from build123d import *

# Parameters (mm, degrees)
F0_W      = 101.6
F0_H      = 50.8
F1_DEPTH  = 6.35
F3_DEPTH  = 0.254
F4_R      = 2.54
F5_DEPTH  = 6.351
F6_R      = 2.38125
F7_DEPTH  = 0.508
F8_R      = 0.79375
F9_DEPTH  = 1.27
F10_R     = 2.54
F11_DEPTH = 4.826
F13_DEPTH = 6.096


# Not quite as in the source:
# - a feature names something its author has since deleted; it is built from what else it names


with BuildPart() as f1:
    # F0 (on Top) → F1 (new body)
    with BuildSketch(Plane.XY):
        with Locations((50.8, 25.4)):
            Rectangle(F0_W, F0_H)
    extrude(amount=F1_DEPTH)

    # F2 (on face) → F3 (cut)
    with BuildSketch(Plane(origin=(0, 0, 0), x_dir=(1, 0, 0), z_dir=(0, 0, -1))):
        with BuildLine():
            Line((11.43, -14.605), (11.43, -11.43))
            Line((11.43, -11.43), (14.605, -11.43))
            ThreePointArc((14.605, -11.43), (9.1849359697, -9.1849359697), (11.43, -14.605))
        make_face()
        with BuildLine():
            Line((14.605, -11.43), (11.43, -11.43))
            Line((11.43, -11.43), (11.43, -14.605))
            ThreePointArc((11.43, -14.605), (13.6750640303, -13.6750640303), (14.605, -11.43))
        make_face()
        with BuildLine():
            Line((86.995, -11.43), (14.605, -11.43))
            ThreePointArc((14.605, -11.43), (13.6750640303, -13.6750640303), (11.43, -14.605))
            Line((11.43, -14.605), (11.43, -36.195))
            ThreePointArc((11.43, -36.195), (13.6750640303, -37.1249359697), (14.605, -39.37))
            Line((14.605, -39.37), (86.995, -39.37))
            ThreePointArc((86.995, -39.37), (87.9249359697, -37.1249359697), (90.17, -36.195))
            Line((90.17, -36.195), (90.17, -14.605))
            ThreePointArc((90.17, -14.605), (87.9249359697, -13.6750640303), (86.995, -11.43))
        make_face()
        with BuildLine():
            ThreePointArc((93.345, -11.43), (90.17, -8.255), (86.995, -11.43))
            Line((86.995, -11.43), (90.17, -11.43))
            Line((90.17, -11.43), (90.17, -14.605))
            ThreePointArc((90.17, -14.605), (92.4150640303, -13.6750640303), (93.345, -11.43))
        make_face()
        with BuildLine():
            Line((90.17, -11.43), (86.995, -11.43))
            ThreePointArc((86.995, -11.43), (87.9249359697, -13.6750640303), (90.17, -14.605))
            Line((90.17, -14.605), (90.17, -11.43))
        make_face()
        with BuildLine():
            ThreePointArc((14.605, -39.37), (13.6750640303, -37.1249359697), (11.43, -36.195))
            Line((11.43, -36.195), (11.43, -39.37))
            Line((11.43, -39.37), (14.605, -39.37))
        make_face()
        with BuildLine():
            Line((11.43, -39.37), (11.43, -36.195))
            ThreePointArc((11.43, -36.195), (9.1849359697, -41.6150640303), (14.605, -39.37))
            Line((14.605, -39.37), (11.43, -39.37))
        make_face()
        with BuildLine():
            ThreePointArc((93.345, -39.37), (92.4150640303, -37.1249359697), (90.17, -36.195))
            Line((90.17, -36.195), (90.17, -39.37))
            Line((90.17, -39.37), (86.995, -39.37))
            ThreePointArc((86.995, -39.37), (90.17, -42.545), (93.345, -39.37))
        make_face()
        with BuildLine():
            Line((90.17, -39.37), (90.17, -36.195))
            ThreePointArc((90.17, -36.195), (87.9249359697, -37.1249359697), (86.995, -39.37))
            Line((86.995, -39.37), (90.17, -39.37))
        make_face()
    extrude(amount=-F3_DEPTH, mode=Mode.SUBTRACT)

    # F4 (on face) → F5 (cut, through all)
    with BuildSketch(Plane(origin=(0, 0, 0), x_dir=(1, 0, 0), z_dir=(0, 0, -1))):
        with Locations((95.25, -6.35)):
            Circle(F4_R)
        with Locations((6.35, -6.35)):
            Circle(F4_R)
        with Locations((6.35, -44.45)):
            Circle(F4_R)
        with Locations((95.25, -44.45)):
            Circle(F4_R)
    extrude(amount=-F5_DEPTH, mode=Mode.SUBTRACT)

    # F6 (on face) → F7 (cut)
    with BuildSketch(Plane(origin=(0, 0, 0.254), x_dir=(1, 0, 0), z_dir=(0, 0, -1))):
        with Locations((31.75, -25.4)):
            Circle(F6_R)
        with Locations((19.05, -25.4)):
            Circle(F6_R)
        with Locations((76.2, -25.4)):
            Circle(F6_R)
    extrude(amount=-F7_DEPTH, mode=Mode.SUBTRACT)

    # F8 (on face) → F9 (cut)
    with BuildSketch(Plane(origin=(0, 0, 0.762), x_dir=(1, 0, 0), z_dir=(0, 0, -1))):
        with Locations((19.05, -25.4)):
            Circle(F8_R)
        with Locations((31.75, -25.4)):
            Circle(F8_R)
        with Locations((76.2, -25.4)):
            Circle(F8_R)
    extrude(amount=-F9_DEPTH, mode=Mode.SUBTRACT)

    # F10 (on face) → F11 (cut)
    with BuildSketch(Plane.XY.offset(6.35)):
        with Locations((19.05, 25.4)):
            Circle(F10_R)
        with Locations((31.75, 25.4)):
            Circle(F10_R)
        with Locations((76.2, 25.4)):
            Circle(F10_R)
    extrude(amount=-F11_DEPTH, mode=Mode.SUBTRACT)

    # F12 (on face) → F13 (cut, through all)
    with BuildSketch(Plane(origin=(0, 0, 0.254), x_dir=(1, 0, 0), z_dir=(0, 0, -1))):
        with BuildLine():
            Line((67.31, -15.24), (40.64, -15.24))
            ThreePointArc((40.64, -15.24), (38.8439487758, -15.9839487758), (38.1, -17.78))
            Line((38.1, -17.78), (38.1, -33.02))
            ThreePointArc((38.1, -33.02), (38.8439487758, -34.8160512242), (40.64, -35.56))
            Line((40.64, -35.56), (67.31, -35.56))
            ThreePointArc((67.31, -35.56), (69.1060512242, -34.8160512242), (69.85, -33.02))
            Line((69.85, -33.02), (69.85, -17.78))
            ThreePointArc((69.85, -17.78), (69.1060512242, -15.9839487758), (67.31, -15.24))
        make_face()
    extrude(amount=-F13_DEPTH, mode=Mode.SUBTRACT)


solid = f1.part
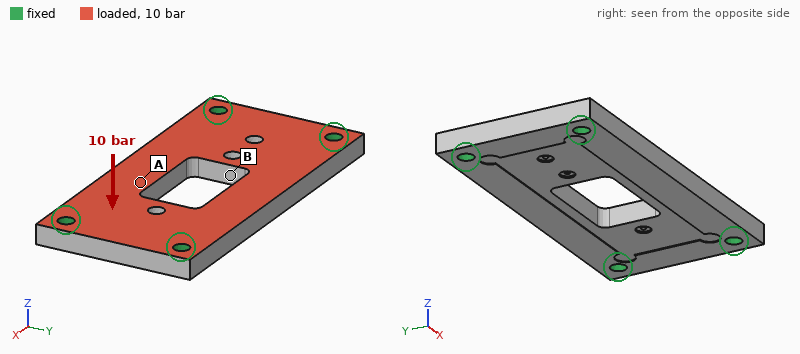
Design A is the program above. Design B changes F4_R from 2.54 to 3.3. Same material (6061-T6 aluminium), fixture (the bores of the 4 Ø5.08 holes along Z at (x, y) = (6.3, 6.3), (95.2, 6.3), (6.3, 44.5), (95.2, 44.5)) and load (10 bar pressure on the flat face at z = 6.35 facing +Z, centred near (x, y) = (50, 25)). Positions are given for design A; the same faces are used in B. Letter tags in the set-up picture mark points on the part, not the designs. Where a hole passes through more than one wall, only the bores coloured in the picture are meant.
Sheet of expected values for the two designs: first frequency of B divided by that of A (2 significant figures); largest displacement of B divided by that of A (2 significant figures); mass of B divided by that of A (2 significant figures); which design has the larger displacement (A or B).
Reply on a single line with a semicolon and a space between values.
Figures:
1.1; 0.89; 0.99; A
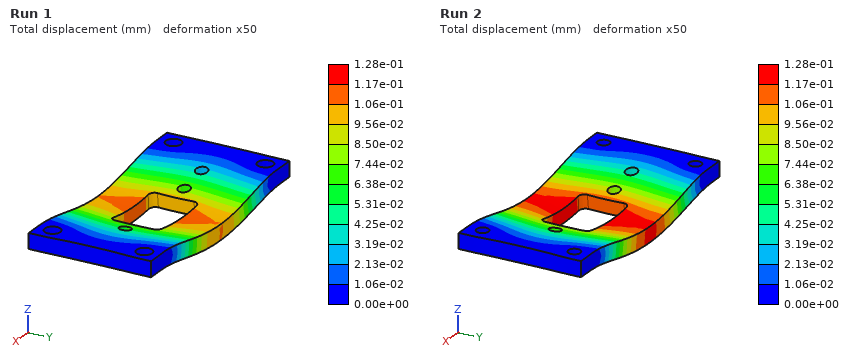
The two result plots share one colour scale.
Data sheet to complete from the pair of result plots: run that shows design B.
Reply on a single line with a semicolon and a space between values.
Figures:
Run 1
